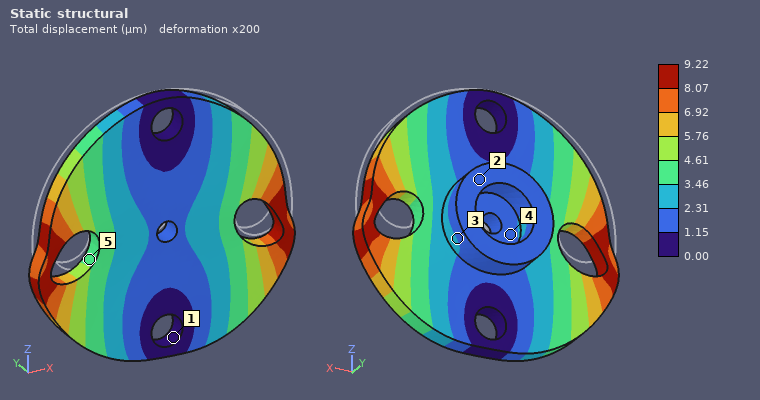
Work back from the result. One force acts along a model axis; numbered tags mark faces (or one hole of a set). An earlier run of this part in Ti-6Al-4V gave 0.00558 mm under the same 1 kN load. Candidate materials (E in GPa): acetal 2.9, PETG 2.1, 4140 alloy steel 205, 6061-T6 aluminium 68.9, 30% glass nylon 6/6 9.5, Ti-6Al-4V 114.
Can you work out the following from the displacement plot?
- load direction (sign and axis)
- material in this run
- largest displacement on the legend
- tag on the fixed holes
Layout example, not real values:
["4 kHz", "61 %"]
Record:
["-Z", "6061-T6 aluminium", "9.22 µm", "1"]
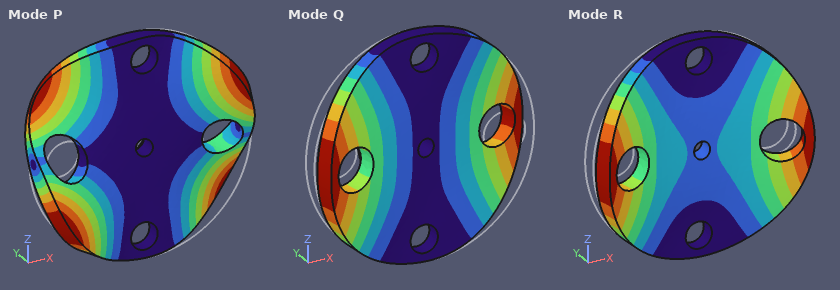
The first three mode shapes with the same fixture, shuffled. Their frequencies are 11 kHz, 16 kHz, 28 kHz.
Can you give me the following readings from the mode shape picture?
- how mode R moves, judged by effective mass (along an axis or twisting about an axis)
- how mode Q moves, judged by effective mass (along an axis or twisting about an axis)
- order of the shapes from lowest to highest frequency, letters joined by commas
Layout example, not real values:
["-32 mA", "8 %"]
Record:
["along Y", "twisting about Z", "Q, R, P"]
